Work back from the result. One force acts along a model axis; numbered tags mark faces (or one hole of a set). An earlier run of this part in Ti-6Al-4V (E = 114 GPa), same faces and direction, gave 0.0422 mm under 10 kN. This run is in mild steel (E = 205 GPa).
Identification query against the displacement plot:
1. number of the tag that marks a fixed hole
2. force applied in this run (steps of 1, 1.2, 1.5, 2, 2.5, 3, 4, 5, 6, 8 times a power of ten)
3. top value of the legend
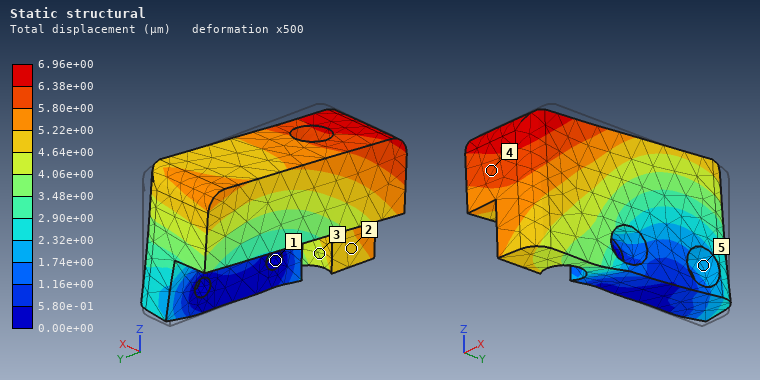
1
3 kN
6.96e+00 µm
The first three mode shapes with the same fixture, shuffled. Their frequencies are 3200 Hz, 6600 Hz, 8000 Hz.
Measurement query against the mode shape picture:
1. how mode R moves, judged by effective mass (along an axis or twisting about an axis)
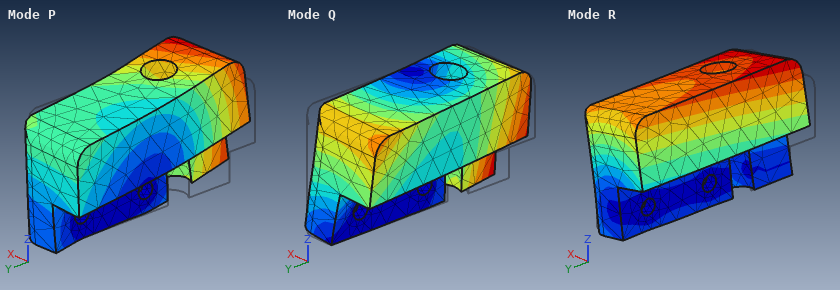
along X
